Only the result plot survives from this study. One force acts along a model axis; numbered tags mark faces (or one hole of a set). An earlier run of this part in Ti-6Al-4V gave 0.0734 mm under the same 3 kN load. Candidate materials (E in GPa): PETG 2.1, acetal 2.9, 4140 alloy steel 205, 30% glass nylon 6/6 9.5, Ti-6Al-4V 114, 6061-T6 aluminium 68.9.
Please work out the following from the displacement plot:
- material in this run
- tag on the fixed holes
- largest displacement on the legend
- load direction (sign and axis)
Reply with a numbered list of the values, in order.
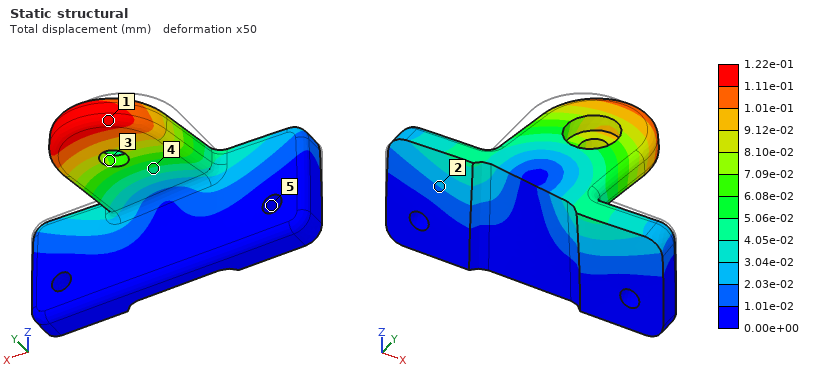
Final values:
1. 6061-T6 aluminium
2. 5
3. 1.22e-01 mm
4. +X
